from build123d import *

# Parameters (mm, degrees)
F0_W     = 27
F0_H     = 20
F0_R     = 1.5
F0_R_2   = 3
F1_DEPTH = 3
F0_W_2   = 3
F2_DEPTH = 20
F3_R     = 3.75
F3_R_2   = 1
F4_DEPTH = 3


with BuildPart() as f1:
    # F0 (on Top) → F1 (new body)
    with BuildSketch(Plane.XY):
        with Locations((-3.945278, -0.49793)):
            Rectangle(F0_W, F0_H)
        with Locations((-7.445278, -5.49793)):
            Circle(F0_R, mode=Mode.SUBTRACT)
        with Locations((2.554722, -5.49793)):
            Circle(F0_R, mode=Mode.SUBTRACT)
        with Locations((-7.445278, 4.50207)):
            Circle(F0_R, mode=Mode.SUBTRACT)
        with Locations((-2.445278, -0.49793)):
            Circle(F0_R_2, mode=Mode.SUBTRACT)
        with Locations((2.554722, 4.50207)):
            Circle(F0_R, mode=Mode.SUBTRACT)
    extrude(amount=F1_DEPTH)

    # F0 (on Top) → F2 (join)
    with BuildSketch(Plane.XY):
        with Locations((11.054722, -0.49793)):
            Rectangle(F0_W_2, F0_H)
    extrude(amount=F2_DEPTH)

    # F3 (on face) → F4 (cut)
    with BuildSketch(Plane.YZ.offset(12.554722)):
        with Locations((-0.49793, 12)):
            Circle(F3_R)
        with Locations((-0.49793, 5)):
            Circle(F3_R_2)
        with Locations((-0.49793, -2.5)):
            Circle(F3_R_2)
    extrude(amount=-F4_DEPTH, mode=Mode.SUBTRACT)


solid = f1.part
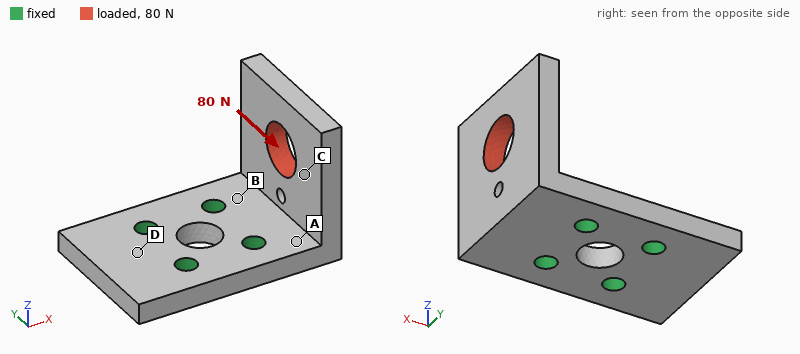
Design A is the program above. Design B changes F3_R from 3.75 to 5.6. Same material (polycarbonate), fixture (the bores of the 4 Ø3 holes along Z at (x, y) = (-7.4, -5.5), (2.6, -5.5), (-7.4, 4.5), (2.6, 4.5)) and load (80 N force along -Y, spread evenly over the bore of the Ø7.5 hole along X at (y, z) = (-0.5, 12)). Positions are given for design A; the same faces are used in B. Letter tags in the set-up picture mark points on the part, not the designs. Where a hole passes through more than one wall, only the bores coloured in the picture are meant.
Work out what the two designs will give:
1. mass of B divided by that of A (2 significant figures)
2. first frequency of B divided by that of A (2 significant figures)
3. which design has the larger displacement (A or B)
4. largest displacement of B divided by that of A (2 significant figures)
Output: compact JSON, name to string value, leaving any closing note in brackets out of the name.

{"mass of B divided by that of A": "0.94", "first frequency of B divided by that of A": "1.0", "which design has the larger displacement": "B", "largest displacement of B divided by that of A": "1.2"}
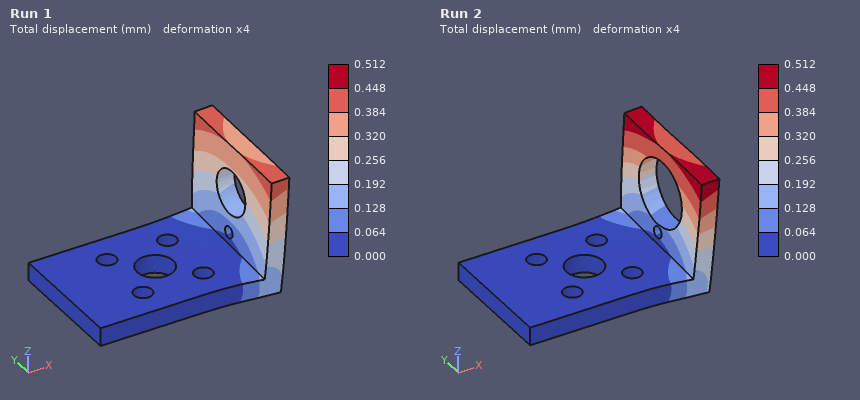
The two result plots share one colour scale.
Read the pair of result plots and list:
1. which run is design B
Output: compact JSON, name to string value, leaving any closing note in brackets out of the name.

{"which run is design B": "Run 2"}
